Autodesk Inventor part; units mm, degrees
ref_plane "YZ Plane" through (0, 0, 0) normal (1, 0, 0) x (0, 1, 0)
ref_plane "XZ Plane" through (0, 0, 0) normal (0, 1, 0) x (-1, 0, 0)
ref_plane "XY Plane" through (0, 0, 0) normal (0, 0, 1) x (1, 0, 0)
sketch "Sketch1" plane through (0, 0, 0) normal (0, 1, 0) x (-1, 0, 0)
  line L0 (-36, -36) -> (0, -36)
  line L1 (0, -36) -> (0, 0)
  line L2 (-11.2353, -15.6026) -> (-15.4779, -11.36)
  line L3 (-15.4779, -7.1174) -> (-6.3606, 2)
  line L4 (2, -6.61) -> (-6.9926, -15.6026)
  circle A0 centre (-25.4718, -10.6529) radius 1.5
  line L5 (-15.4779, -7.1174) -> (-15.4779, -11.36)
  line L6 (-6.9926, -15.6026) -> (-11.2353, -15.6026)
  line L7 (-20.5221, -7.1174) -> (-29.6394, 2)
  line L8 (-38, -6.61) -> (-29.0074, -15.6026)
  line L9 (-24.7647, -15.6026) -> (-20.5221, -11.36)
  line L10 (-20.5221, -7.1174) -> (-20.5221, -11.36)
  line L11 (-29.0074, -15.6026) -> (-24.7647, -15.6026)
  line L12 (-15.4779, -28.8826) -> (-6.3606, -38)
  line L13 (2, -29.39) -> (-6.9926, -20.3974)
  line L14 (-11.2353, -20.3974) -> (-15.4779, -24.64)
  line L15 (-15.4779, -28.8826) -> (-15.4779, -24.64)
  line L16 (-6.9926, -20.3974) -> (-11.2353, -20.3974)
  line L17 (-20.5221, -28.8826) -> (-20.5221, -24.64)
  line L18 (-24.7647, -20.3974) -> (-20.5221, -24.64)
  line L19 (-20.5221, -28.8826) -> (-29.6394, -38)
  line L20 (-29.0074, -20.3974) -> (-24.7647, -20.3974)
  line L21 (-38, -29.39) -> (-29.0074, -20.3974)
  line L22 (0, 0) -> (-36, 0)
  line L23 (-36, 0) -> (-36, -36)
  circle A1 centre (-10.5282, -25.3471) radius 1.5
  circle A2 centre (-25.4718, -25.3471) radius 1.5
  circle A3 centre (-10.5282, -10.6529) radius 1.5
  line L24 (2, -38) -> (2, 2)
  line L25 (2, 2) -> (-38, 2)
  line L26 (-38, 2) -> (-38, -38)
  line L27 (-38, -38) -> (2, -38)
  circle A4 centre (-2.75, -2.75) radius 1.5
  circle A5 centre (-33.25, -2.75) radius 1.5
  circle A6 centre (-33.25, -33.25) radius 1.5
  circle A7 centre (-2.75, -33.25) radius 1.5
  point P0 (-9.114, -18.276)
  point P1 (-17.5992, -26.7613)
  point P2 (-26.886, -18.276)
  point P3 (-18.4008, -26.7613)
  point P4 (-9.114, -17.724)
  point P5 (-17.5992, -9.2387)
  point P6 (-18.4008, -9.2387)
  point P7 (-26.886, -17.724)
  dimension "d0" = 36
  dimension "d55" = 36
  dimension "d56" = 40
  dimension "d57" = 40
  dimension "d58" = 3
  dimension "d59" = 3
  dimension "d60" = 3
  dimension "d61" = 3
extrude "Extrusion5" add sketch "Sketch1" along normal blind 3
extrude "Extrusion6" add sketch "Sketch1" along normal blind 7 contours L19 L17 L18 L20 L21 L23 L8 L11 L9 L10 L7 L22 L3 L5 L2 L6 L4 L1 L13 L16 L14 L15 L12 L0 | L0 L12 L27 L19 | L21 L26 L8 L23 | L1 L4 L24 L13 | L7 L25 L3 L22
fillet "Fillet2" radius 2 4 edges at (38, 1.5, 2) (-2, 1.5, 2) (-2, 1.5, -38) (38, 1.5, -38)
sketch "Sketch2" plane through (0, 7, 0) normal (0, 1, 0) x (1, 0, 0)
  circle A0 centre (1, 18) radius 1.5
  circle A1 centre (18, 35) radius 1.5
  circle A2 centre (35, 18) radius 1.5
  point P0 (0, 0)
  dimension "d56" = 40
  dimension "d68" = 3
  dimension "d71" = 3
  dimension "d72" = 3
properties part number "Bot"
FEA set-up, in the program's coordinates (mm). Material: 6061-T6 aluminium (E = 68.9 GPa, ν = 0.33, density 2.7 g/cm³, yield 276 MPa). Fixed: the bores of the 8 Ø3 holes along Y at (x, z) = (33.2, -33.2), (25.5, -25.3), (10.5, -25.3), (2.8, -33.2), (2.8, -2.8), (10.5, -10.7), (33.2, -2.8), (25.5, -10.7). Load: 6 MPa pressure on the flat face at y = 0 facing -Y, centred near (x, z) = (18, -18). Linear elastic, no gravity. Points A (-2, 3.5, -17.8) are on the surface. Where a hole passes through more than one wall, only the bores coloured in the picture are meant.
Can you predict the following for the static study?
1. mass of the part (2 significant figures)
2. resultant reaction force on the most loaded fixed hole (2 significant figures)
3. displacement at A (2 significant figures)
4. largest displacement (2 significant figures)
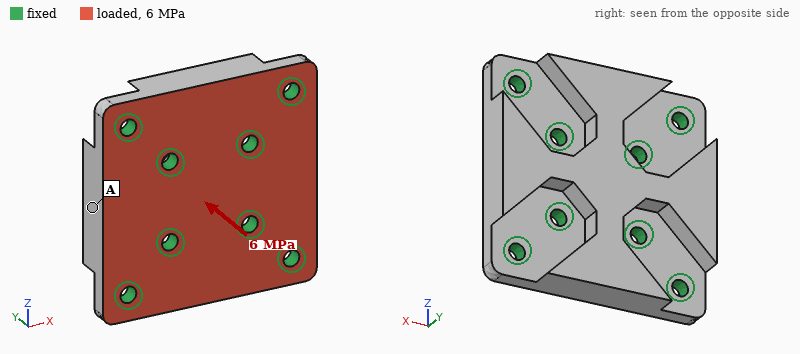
20 g
1.3 kN
18 µm
19 µm
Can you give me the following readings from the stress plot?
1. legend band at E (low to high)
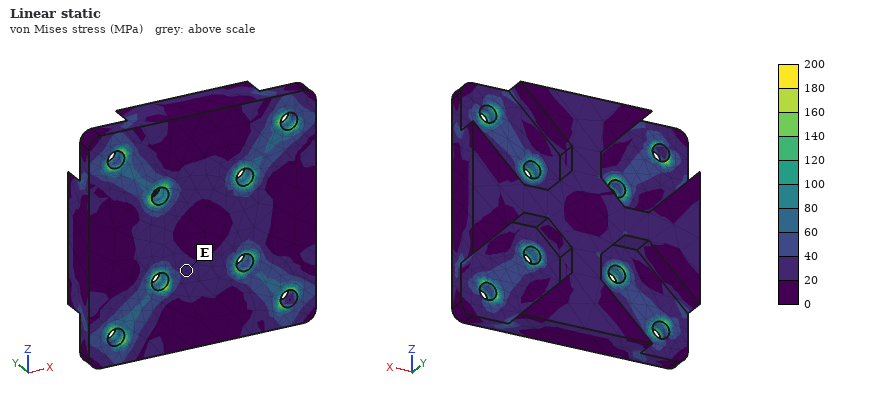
20 to 40 MPa
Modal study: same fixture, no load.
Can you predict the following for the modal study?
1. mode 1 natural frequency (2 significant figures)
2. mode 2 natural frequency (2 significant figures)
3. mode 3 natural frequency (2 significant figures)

24 kHz
25 kHz
25 kHz
